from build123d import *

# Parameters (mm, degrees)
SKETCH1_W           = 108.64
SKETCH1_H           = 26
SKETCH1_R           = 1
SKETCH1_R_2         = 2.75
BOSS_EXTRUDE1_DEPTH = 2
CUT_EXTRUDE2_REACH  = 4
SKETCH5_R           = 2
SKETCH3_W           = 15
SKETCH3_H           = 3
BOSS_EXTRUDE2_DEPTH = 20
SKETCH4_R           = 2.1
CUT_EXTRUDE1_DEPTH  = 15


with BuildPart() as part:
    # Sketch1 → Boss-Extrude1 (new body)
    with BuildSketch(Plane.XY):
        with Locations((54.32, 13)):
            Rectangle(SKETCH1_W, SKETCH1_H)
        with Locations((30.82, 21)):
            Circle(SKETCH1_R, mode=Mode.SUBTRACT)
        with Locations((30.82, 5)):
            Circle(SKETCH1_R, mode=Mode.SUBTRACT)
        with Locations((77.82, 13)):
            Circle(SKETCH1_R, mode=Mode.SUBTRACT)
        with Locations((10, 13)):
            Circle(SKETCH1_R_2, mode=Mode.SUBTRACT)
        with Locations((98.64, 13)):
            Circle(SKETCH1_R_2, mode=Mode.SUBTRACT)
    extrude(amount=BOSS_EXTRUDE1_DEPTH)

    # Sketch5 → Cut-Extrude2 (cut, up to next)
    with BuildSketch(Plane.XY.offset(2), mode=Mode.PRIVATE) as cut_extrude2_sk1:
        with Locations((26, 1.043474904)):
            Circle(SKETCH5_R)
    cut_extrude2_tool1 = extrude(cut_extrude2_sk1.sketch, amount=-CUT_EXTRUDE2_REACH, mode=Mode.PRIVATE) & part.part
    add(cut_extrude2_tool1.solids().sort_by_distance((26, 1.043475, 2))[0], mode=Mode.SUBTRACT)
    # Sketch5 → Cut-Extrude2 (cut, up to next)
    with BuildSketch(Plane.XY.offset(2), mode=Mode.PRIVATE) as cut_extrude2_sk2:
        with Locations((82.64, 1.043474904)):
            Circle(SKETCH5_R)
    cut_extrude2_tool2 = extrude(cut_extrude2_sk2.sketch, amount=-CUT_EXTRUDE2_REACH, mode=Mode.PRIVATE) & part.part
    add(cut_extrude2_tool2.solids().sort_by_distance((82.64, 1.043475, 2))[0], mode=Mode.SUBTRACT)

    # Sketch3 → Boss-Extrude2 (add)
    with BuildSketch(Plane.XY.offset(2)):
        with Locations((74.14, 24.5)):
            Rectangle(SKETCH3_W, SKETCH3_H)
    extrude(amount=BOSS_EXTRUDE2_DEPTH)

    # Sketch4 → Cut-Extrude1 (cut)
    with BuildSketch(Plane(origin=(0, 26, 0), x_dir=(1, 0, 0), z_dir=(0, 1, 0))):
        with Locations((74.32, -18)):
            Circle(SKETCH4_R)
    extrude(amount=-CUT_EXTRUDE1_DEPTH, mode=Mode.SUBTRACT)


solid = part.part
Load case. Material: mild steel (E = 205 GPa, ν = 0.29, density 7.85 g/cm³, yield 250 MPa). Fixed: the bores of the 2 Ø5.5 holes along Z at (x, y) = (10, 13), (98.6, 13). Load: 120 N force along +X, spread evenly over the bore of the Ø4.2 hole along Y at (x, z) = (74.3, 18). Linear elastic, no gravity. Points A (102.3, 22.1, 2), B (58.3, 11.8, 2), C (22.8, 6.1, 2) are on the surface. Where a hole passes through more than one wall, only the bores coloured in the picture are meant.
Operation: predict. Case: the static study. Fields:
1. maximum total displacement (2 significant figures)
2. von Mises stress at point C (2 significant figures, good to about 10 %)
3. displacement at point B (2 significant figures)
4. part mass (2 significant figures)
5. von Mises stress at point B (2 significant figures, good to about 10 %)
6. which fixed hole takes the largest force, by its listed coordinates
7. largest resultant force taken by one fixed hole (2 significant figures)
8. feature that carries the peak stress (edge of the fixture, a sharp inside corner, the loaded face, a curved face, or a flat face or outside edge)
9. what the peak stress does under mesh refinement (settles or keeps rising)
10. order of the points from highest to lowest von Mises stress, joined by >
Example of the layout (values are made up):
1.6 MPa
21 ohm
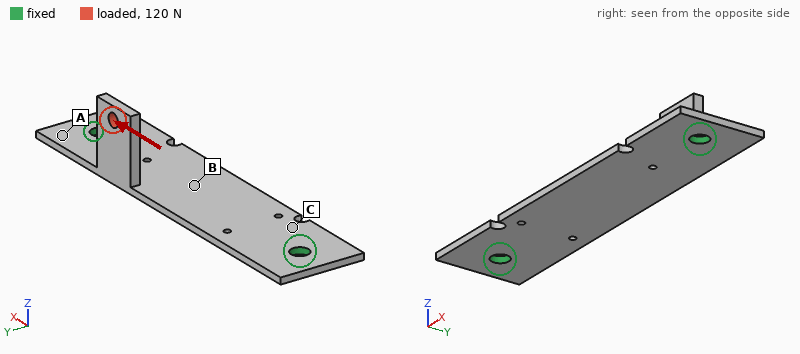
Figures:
0.12 mm
21 MPa
0.060 mm
50 g
37 MPa
(98.6, 13)
88 N
a sharp inside corner
keeps rising
B > C > A
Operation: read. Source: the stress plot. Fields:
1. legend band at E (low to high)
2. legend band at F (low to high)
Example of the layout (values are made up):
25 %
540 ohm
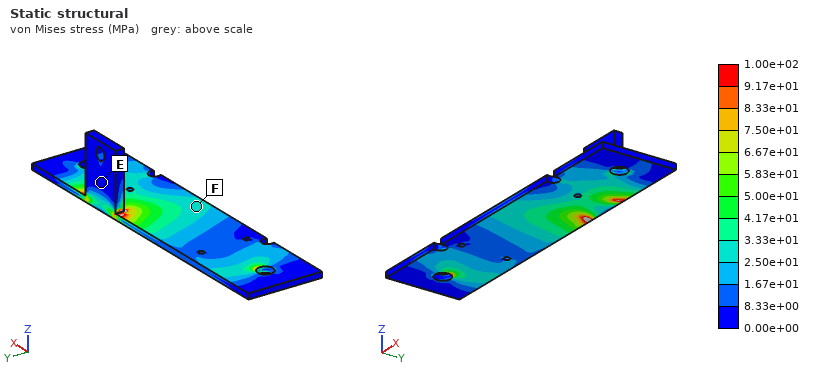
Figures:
0.00e+00 to 8.33e+00 MPa
2.50e+01 to 3.33e+01 MPa
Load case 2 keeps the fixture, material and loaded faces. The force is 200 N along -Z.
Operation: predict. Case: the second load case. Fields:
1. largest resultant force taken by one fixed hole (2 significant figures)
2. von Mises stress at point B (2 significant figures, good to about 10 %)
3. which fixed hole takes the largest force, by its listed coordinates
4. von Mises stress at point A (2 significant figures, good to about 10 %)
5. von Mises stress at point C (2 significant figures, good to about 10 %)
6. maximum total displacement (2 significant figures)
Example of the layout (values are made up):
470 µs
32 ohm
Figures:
160 N
55 MPa
(98.6, 13)
58 MPa
43 MPa
0.23 mm
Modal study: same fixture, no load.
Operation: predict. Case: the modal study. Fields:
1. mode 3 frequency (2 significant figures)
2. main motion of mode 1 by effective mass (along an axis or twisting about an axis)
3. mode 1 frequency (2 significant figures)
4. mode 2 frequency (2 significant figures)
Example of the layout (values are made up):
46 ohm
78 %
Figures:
3600 Hz
along Z
1200 Hz
1800 Hz
